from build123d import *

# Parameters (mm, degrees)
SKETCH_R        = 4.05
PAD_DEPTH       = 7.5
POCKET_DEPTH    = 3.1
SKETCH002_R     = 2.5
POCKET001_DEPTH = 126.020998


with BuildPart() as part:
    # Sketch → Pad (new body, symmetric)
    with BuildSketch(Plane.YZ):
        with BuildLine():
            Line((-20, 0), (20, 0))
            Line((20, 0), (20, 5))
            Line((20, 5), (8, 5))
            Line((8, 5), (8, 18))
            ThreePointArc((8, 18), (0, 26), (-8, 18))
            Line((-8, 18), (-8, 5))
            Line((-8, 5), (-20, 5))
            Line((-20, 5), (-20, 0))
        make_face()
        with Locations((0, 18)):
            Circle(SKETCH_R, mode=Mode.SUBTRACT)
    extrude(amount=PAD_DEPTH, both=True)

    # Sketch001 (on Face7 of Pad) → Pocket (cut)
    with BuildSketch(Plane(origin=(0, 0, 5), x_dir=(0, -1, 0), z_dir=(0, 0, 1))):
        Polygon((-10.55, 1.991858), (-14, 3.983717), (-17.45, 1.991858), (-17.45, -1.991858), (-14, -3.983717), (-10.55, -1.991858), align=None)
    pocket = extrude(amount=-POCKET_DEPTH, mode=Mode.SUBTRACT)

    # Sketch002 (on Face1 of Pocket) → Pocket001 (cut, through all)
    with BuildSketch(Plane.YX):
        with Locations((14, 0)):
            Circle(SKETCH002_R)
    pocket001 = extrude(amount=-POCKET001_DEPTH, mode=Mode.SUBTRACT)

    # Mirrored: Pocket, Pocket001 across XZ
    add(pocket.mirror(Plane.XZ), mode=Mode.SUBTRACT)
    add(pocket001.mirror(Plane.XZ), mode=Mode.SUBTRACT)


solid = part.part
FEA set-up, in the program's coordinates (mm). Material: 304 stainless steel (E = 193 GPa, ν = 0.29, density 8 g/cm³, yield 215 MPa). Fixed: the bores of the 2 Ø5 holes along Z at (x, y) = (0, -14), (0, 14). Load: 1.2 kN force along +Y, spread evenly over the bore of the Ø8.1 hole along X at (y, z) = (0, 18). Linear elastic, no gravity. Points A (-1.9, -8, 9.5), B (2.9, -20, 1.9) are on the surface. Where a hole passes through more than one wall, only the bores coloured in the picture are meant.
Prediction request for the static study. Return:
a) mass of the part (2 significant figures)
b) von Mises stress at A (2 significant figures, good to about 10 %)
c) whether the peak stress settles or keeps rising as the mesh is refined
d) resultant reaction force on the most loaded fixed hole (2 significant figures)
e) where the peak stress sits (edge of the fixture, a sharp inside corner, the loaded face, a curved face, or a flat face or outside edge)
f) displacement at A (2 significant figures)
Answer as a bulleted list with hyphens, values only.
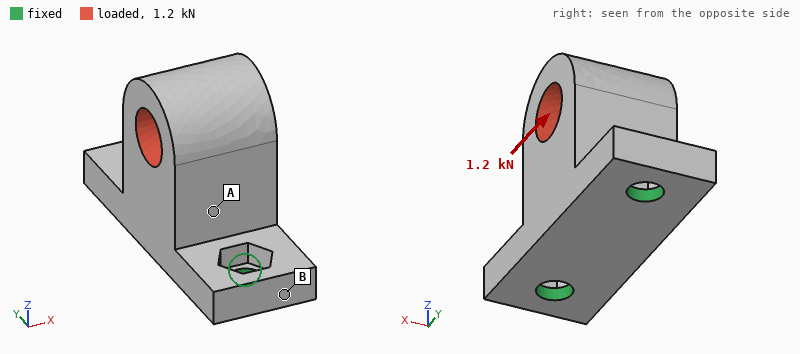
- 52 g
- 22 MPa
- keeps rising
- 1.0 kN
- edge of the fixture
- 4.2 µm
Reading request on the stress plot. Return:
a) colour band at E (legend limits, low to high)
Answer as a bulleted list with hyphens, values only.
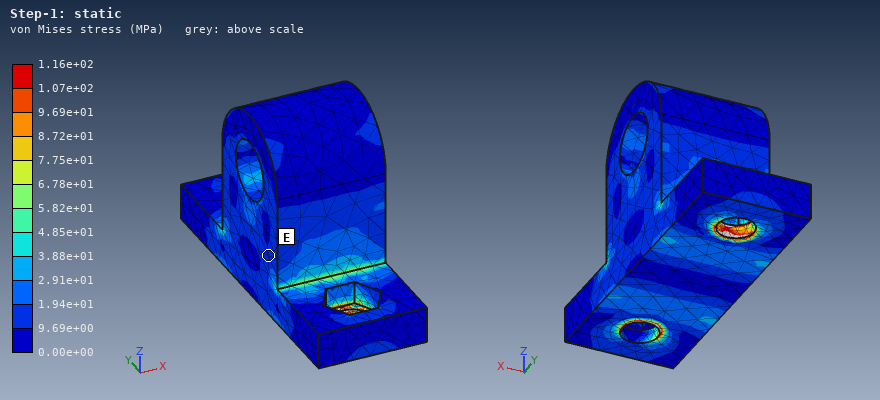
- 9.69e+00 to 1.94e+01 MPa
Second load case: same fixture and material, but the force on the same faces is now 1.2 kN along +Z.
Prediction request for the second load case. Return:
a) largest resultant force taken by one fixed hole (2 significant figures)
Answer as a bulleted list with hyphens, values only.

- 750 N
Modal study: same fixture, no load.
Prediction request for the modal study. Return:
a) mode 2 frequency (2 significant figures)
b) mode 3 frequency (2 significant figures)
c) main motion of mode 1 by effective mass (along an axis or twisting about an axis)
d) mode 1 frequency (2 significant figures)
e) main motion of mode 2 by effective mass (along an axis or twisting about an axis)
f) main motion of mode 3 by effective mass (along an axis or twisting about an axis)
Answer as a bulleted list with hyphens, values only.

- 13 kHz
- 16 kHz
- along X
- 4500 Hz
- along Y
- along Z
